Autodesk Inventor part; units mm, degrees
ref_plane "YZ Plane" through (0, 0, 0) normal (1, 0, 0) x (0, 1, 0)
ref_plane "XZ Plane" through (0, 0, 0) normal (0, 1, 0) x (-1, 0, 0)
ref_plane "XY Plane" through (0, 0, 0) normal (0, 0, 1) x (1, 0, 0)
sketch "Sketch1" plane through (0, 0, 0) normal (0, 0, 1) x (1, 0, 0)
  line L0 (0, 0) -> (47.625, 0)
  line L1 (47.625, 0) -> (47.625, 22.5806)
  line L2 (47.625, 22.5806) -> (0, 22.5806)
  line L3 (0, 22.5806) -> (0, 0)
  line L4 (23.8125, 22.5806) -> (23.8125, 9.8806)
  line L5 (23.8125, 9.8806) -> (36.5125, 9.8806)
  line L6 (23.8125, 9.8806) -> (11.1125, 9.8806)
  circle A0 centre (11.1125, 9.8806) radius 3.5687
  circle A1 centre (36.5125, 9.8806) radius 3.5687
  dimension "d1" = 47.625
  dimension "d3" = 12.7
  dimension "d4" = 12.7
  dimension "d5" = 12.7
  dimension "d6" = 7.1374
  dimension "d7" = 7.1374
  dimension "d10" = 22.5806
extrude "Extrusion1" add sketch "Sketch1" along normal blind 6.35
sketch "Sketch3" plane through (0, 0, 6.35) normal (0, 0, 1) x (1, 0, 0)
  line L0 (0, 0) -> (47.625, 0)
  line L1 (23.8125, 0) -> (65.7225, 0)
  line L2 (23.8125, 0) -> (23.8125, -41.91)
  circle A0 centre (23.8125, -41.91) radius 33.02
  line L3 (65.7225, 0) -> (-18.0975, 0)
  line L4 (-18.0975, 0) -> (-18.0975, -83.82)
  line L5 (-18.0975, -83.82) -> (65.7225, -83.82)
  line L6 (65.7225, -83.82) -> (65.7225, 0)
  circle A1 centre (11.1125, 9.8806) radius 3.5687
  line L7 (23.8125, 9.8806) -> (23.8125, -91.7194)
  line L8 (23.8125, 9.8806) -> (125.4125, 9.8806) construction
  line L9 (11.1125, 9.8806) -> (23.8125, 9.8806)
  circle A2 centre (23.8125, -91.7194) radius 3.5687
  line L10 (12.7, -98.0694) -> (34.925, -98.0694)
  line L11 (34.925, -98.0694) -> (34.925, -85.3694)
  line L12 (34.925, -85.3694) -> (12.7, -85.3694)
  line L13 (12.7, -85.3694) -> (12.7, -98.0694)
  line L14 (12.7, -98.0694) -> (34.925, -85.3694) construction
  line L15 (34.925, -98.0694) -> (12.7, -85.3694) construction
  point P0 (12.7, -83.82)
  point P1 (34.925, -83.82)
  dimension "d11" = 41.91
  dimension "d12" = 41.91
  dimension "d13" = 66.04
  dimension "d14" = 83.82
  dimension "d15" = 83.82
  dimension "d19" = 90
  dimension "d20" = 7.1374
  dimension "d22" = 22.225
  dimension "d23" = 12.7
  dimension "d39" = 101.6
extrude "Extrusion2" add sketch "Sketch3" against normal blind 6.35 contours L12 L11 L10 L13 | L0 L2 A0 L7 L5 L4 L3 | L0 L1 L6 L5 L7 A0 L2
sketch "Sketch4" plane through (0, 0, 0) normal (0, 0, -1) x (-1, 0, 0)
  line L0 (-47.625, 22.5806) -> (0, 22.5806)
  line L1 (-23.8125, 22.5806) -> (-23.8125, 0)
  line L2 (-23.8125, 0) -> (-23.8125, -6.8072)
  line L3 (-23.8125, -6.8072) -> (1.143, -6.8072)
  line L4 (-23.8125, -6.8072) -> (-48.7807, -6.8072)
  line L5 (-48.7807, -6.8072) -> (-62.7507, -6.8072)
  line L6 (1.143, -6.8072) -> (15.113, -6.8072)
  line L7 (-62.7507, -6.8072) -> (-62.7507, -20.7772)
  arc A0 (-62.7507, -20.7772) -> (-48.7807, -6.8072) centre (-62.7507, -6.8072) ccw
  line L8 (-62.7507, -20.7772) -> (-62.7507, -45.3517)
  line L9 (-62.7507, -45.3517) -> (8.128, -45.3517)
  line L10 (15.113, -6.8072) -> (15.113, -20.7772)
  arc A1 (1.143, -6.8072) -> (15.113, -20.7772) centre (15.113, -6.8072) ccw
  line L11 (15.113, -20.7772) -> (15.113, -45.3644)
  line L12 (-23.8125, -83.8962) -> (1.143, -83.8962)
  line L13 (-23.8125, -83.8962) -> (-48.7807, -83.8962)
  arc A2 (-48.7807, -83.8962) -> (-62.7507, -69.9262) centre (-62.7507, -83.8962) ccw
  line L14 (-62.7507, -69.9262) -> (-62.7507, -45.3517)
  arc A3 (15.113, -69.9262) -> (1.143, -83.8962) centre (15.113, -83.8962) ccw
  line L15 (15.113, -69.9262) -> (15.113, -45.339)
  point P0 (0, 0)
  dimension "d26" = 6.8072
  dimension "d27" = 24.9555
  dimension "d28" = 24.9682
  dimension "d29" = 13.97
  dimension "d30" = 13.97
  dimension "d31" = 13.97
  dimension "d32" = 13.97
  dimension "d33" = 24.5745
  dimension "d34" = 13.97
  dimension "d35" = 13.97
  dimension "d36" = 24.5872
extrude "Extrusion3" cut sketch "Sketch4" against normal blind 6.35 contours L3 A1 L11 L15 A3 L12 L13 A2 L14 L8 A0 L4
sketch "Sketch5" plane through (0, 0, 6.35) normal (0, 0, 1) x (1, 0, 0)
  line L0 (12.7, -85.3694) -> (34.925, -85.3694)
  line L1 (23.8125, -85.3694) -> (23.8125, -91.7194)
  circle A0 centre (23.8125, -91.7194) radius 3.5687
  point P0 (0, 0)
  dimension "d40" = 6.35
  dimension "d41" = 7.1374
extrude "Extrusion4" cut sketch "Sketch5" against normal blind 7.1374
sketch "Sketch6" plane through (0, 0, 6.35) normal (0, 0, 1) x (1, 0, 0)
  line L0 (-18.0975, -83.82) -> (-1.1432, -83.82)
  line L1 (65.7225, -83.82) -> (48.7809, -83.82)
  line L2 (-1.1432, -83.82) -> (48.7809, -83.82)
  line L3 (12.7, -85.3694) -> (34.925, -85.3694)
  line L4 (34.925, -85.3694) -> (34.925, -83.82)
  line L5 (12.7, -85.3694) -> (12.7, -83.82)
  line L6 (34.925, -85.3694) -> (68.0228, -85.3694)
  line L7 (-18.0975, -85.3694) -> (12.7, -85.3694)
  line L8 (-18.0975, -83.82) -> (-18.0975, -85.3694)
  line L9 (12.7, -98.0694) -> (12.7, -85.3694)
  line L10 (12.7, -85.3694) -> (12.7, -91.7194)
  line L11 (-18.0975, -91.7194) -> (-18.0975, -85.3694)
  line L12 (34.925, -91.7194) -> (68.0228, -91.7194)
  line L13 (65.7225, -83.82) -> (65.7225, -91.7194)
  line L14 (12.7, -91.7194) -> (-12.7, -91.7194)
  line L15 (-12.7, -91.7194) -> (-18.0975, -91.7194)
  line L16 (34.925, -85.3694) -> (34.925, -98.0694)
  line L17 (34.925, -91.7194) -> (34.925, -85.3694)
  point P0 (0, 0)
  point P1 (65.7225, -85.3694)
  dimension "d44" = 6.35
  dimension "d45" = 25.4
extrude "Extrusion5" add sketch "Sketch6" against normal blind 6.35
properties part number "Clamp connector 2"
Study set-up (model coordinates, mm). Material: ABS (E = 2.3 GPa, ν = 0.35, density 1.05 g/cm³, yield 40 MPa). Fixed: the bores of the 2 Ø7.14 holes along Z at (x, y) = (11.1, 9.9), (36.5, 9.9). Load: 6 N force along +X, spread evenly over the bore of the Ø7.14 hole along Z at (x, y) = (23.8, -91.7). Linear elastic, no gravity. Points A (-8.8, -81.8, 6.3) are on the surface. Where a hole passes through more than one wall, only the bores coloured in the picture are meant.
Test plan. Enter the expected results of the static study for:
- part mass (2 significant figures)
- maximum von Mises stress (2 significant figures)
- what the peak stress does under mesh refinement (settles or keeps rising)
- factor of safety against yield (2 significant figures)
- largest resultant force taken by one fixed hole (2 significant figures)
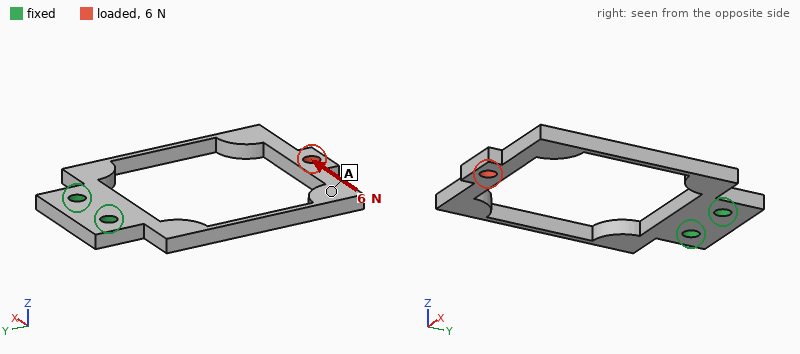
23 g
7.6 MPa
settles
5.3
18 N
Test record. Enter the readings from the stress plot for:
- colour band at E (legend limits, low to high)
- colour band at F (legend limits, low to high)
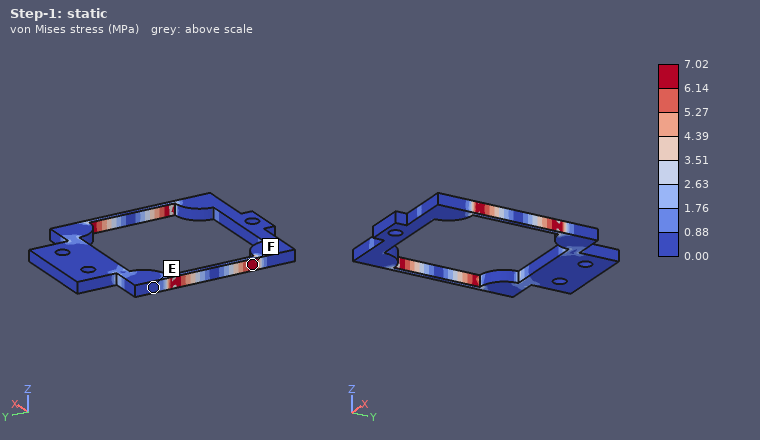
0.00 to 0.88 MPa
6.14 to 7.02 MPa
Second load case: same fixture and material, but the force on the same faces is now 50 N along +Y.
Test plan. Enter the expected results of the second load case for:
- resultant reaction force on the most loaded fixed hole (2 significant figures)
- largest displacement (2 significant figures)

41 N
0.73 mm
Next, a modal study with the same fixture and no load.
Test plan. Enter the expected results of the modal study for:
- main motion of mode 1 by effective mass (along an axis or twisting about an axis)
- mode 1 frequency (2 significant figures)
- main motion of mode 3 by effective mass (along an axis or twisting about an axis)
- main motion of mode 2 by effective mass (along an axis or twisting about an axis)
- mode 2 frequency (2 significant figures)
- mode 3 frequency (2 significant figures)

along Z
74 Hz
twisting about Y
along X
110 Hz
190 Hz
